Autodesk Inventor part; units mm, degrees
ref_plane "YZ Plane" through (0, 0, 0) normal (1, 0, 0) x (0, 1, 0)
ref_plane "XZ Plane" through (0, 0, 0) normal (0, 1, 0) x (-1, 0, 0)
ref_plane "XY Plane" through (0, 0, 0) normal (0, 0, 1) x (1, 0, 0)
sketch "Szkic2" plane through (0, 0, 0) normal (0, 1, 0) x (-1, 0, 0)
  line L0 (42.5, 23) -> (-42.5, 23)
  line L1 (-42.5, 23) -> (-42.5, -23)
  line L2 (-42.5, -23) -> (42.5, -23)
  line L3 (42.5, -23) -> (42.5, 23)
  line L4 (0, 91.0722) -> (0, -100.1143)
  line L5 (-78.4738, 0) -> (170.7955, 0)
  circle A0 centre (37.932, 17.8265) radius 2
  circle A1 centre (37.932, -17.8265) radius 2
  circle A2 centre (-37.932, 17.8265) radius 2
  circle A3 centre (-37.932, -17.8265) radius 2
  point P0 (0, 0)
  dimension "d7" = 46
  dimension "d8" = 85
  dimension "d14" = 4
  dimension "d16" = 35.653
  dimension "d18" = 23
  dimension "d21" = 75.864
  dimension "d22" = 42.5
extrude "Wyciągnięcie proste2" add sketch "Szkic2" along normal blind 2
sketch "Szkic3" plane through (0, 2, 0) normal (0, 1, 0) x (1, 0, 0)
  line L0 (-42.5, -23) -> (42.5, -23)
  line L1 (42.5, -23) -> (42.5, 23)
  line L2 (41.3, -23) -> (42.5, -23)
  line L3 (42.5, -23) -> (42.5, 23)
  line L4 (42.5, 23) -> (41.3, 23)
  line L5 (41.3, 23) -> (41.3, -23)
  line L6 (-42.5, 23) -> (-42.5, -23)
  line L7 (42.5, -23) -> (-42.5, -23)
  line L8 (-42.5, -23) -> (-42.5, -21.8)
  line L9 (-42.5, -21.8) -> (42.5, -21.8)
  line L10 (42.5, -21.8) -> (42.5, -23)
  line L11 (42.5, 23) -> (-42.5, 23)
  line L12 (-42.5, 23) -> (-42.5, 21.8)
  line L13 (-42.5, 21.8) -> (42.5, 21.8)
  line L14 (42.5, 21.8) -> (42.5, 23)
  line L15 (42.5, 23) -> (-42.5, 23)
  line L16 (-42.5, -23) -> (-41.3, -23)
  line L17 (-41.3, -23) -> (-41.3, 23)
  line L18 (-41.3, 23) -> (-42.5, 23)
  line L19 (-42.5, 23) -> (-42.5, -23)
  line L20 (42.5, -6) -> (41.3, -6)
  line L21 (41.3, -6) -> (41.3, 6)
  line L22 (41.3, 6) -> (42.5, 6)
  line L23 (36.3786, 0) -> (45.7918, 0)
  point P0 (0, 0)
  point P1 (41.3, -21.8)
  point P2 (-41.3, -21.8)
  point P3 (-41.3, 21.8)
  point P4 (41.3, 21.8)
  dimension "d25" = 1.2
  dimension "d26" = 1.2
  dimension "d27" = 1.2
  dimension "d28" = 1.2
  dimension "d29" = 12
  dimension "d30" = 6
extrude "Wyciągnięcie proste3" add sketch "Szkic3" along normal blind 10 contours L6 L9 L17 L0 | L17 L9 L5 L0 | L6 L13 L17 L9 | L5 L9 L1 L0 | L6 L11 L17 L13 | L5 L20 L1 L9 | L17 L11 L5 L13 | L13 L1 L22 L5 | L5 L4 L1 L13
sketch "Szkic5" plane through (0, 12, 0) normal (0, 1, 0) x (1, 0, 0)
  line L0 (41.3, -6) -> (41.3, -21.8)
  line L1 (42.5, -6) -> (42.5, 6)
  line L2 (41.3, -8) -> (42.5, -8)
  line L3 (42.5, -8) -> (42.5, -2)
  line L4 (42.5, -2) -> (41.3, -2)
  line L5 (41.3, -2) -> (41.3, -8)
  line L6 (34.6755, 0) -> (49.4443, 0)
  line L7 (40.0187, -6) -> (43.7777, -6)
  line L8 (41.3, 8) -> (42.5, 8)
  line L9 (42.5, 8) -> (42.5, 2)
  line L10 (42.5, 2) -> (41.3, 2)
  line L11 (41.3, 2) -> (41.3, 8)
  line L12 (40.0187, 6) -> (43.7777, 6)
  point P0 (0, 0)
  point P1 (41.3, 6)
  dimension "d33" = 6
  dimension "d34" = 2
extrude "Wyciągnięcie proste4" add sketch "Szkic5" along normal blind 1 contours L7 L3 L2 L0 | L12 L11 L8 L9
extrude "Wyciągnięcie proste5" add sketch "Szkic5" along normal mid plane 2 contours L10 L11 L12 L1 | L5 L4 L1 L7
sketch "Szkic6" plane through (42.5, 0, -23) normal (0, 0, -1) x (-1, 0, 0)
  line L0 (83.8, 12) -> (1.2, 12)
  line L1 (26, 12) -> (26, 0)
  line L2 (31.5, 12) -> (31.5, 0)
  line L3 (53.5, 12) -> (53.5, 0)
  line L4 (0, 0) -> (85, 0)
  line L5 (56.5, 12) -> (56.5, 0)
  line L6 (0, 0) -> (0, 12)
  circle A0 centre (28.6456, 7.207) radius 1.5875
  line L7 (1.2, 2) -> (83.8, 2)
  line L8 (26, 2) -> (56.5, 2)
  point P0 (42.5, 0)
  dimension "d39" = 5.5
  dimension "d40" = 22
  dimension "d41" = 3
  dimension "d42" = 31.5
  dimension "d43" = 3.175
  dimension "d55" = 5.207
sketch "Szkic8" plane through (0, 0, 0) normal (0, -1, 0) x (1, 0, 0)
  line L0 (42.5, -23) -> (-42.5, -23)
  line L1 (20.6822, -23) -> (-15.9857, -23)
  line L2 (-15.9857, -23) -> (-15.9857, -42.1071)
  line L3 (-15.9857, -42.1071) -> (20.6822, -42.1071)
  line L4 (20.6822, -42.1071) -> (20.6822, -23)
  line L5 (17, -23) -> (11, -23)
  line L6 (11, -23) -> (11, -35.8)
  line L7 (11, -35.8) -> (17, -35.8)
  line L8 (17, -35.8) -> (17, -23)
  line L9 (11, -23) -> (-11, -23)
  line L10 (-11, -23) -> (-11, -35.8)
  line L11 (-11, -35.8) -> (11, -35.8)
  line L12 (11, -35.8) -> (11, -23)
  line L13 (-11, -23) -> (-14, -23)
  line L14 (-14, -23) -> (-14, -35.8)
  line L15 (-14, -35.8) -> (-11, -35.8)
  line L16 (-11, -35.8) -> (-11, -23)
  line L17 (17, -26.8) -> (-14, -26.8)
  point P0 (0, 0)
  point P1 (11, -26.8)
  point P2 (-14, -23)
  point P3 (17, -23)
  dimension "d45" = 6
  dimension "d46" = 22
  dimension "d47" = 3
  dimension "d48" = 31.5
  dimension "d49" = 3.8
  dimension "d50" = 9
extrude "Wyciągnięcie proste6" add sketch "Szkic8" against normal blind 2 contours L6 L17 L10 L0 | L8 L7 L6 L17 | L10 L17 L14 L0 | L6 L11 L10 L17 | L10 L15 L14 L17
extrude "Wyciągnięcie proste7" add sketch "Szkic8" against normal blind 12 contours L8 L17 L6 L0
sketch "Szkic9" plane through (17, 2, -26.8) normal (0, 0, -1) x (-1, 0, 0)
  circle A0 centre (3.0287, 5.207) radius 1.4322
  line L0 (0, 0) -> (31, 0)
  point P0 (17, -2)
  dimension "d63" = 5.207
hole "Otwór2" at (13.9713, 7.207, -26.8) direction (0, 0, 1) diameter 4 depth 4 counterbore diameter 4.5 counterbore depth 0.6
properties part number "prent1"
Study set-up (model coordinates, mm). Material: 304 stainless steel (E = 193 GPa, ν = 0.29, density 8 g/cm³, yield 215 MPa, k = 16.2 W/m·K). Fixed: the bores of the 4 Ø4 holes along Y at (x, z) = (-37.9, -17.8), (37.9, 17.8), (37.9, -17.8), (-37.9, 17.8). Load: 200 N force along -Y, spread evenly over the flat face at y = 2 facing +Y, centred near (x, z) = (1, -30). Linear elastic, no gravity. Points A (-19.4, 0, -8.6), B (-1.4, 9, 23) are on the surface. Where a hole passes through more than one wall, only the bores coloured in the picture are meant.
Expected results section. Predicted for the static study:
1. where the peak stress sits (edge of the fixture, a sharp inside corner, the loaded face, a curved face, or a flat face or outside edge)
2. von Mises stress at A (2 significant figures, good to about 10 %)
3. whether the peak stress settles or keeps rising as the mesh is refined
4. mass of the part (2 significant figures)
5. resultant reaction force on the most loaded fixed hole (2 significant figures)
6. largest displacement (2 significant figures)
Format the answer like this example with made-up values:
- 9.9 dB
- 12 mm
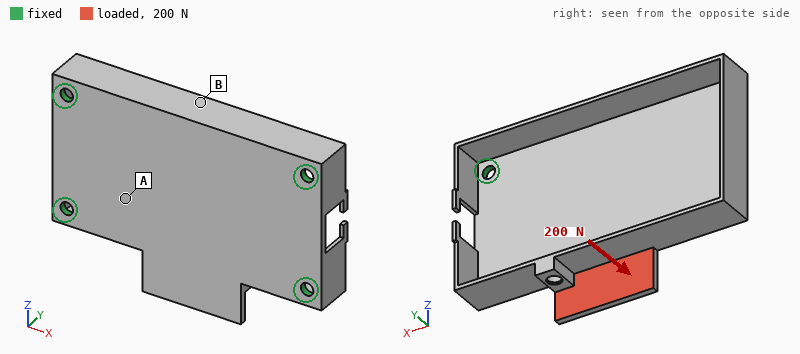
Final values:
- edge of the fixture
- 14 MPa
- keeps rising
- 93 g
- 210 N
- 76 µm
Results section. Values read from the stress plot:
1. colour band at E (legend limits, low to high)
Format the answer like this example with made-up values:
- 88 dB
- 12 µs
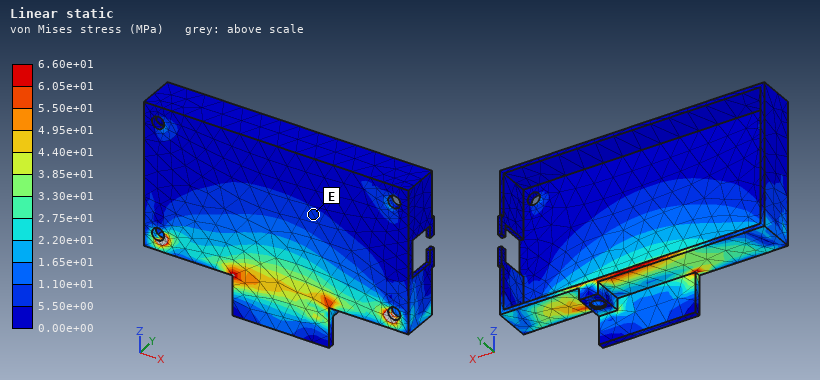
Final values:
- 5.50e+00 to 1.10e+01 MPa
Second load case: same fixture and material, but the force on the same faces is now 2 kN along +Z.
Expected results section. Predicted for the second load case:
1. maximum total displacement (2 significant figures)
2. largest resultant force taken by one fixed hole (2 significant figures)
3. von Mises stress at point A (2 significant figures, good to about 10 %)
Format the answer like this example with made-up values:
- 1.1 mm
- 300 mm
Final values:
- 83 µm
- 690 N
- 22 MPa
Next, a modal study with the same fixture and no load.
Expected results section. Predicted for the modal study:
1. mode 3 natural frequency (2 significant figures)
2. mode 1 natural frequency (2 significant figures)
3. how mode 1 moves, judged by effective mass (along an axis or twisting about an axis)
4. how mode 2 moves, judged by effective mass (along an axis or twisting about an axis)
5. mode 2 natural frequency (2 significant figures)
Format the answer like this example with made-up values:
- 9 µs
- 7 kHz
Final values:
- 5600 Hz
- 2900 Hz
- along Y
- along Y
- 3400 Hz
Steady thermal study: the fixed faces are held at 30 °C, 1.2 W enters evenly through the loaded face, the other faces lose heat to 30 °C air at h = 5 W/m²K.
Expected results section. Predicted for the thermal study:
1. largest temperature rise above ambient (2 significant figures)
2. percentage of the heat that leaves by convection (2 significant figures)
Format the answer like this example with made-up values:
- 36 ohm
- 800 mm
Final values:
- 24 K
- 29 %
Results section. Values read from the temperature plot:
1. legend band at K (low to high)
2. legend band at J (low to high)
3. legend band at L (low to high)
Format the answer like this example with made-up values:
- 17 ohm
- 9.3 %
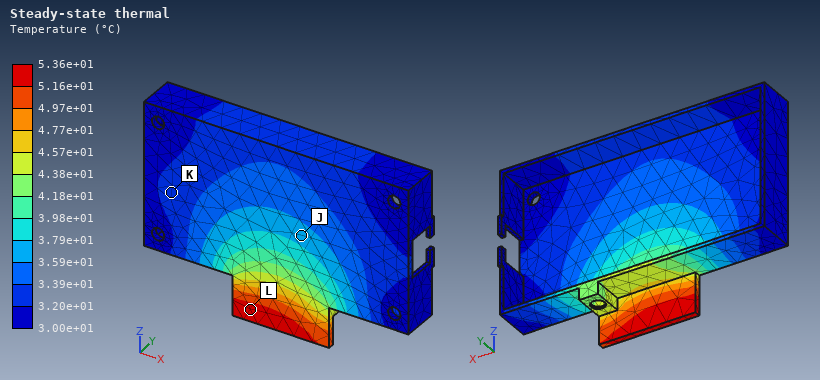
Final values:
- 3.20e+01 to 3.39e+01 °C
- 3.59e+01 to 3.79e+01 °C
- 5.16e+01 to 5.36e+01 °C
